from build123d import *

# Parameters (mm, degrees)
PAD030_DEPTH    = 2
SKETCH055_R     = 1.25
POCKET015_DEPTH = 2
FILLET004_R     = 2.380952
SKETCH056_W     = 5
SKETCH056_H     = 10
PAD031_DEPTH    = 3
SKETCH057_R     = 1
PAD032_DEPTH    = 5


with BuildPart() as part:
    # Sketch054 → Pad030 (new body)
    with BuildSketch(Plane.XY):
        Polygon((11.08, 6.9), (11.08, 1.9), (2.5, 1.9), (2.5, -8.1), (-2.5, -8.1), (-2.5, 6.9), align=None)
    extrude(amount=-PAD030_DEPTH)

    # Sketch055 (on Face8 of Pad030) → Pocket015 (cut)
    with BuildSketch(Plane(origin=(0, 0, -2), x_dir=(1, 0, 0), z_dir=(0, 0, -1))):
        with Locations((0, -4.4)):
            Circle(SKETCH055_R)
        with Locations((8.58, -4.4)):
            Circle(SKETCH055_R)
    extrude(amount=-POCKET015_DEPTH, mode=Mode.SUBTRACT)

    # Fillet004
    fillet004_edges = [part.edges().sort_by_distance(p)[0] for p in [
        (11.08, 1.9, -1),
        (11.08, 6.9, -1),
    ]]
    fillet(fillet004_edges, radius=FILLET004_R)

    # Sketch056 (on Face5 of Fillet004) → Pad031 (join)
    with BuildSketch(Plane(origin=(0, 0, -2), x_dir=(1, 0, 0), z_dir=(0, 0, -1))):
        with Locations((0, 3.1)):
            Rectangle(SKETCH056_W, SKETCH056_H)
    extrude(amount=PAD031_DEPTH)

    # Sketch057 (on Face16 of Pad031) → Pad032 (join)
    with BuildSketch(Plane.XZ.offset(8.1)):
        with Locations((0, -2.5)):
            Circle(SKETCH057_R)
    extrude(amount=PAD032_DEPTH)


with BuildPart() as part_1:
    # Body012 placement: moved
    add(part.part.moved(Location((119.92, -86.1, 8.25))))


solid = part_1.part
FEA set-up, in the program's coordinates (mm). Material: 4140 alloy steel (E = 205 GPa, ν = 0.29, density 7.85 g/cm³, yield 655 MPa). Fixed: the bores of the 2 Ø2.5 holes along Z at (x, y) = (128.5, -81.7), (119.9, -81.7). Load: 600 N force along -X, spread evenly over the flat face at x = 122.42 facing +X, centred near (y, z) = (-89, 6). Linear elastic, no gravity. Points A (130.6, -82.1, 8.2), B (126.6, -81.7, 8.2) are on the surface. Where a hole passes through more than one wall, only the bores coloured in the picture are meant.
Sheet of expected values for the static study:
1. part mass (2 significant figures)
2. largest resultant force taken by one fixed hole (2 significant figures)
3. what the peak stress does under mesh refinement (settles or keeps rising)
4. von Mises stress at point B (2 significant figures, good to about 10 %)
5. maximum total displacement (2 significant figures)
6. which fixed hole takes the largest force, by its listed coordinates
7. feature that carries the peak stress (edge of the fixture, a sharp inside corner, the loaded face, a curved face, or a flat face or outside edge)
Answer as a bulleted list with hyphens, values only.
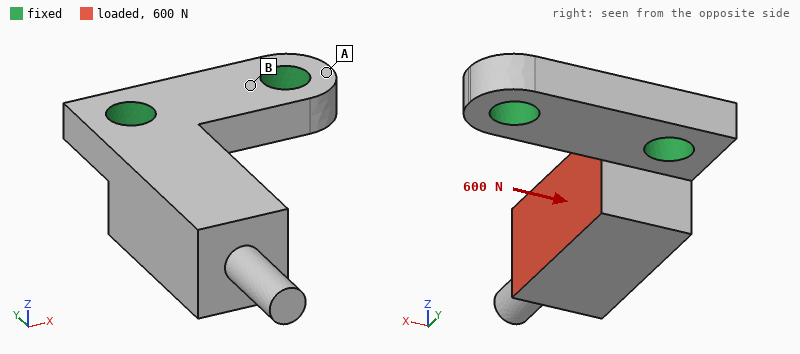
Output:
- 3.0 g
- 460 N
- keeps rising
- 98 MPa
- 53 µm
- (119.9, -81.7)
- a sharp inside corner
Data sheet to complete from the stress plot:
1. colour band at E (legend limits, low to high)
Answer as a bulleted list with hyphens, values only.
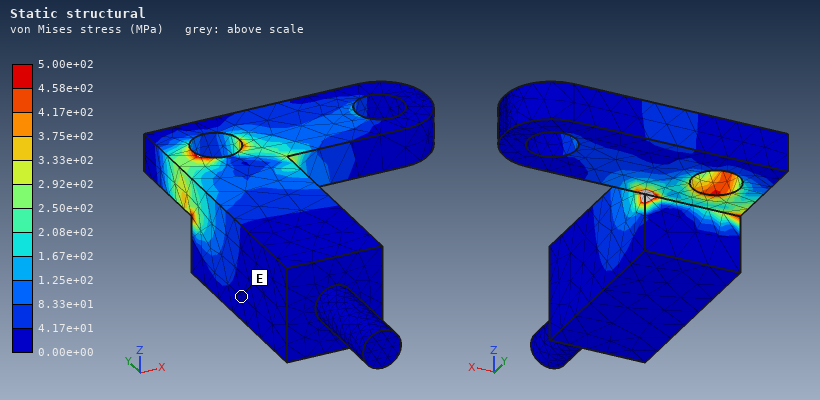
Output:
- 0.00e+00 to 4.17e+01 MPa
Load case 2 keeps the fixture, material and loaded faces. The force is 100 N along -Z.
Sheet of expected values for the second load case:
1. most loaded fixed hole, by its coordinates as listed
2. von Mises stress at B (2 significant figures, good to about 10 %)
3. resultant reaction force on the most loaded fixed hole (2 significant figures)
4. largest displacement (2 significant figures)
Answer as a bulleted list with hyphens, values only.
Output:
- (119.9, -81.7)
- 17 MPa
- 96 N
- 33 µm
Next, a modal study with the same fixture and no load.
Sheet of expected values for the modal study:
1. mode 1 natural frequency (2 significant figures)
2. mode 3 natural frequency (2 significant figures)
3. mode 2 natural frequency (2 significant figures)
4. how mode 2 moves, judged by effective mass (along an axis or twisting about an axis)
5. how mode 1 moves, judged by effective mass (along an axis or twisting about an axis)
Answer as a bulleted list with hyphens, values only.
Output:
- 7900 Hz
- 34 kHz
- 15 kHz
- along X
- along Z
